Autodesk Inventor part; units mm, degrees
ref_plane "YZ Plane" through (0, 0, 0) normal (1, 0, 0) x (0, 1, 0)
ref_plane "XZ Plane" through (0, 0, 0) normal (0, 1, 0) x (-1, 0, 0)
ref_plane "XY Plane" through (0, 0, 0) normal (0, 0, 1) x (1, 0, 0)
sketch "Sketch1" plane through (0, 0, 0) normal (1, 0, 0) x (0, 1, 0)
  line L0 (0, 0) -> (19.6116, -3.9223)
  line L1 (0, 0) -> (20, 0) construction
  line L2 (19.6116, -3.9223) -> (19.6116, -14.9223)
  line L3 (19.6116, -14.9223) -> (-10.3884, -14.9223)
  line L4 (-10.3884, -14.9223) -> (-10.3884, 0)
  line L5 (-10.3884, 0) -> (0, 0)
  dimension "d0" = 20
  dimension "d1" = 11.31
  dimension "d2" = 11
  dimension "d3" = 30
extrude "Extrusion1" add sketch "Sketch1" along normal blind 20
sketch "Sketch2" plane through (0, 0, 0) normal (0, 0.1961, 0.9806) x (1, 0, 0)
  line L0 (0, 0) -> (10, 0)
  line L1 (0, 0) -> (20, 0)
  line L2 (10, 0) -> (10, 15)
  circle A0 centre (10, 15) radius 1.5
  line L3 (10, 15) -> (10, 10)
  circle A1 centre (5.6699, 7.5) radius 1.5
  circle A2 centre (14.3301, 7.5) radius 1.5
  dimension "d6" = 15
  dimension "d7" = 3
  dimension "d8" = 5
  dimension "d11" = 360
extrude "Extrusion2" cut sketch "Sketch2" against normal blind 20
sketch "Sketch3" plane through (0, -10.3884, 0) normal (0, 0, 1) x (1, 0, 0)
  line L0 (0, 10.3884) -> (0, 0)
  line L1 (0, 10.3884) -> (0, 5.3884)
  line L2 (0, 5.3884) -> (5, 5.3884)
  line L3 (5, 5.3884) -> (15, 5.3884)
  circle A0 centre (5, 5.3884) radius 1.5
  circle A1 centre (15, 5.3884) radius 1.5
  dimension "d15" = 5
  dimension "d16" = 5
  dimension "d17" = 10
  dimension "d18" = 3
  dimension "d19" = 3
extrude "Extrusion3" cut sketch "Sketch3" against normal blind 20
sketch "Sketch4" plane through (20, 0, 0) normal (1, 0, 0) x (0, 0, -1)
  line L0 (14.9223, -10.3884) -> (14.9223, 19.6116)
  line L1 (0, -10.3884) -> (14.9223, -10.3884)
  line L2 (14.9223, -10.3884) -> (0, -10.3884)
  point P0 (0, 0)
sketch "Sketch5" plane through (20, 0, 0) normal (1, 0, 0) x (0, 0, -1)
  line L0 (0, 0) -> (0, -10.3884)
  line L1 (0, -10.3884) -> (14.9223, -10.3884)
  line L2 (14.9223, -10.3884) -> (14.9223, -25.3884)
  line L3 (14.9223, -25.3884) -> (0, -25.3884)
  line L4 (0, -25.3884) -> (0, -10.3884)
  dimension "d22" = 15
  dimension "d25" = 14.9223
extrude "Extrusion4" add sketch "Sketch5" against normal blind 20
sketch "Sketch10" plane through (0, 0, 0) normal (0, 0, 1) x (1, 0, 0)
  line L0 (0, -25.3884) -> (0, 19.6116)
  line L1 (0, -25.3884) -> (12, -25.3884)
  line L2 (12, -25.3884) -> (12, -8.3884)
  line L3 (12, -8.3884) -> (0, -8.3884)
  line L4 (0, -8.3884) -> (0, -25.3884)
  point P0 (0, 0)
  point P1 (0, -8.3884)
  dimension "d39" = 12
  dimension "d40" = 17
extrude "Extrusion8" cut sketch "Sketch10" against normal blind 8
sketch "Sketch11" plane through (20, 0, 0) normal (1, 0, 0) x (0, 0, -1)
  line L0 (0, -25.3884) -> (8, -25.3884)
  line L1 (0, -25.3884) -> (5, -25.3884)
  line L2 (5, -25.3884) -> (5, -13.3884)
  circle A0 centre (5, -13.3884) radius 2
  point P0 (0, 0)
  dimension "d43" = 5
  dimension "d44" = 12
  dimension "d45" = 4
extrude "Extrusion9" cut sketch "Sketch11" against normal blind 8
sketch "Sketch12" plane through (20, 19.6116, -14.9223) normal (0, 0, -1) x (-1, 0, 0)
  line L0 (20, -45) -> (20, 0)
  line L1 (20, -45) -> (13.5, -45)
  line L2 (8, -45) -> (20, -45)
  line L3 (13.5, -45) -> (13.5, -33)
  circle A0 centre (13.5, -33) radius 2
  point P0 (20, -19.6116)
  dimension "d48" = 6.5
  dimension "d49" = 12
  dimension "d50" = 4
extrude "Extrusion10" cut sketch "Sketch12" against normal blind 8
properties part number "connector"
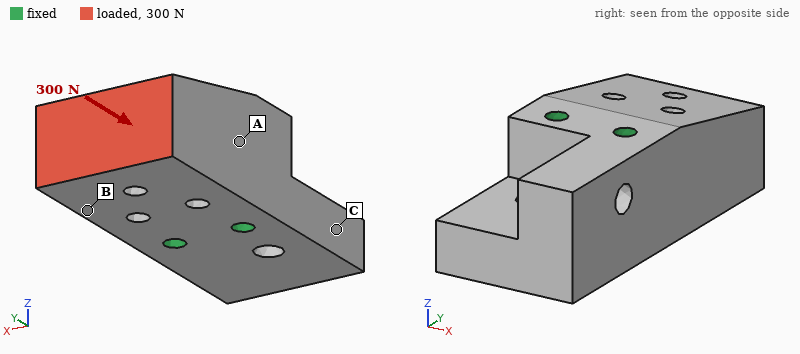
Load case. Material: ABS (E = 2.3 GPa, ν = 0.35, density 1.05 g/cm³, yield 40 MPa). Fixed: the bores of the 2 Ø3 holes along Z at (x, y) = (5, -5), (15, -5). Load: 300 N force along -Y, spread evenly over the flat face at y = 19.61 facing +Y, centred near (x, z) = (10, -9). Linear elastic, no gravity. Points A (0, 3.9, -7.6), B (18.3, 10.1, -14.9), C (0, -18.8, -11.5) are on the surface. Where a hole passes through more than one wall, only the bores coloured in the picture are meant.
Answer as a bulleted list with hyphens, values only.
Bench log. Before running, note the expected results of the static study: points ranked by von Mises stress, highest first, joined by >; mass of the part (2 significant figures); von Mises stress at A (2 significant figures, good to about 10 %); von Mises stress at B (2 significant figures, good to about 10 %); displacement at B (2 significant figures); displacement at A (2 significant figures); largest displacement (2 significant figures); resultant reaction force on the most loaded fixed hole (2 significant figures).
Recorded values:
- B > A > C
- 11 g
- 1.1 MPa
- 1.8 MPa
- 15 µm
- 5.7 µm
- 26 µm
- 150 N
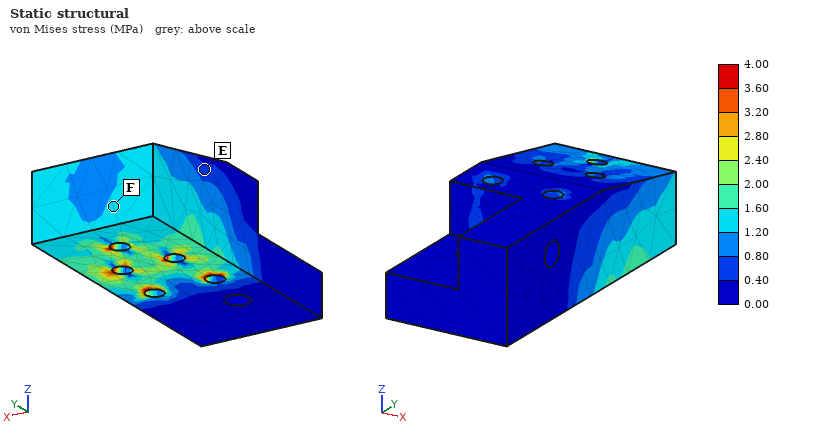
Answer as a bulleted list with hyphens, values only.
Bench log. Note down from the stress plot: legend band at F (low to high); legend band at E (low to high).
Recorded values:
- 1.20 to 1.60 MPa
- 0.40 to 0.80 MPa
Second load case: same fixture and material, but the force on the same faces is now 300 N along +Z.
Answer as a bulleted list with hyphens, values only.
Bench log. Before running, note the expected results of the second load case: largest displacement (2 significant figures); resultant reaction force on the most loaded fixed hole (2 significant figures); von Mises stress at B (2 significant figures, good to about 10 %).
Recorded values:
- 0.21 mm
- 150 N
- 5.8 MPa
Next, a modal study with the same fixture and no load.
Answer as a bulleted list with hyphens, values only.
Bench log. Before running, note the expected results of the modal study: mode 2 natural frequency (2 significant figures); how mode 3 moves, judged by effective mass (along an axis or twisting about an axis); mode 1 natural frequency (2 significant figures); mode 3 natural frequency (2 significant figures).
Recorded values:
- 5200 Hz
- along Z
- 4900 Hz
- 5500 Hz
